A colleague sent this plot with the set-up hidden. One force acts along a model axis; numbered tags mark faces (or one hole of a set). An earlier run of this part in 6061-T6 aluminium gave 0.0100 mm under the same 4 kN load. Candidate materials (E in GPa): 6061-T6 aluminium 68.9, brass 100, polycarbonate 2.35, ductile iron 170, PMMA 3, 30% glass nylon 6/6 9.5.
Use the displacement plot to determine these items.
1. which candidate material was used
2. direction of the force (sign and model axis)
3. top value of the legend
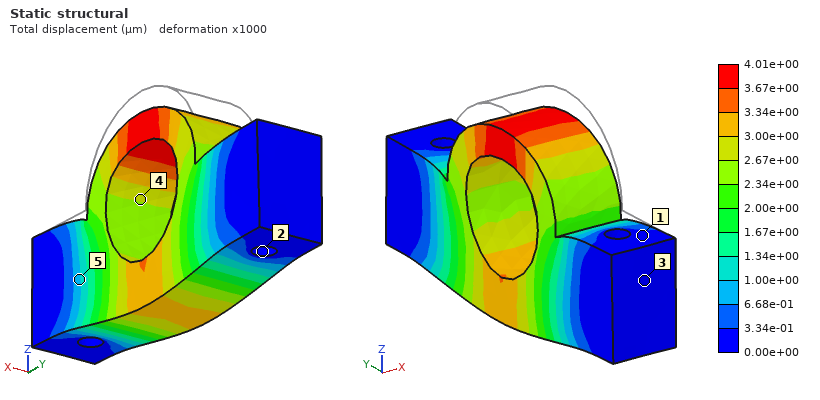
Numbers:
ductile iron
-Z
4.01e+00 µm
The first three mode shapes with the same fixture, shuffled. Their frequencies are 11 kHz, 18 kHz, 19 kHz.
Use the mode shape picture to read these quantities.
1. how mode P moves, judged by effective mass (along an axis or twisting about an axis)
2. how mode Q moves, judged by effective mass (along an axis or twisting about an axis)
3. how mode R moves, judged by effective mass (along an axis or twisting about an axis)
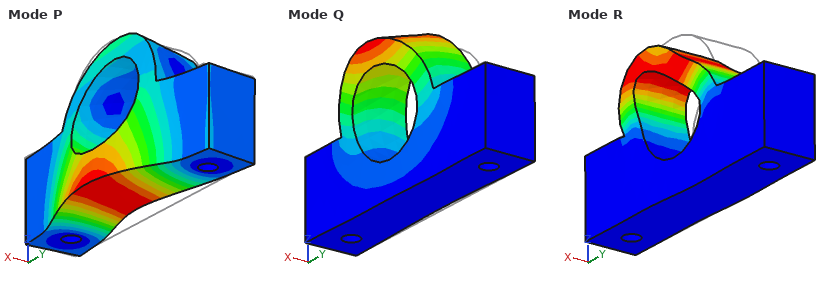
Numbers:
along X
along X
along Y
